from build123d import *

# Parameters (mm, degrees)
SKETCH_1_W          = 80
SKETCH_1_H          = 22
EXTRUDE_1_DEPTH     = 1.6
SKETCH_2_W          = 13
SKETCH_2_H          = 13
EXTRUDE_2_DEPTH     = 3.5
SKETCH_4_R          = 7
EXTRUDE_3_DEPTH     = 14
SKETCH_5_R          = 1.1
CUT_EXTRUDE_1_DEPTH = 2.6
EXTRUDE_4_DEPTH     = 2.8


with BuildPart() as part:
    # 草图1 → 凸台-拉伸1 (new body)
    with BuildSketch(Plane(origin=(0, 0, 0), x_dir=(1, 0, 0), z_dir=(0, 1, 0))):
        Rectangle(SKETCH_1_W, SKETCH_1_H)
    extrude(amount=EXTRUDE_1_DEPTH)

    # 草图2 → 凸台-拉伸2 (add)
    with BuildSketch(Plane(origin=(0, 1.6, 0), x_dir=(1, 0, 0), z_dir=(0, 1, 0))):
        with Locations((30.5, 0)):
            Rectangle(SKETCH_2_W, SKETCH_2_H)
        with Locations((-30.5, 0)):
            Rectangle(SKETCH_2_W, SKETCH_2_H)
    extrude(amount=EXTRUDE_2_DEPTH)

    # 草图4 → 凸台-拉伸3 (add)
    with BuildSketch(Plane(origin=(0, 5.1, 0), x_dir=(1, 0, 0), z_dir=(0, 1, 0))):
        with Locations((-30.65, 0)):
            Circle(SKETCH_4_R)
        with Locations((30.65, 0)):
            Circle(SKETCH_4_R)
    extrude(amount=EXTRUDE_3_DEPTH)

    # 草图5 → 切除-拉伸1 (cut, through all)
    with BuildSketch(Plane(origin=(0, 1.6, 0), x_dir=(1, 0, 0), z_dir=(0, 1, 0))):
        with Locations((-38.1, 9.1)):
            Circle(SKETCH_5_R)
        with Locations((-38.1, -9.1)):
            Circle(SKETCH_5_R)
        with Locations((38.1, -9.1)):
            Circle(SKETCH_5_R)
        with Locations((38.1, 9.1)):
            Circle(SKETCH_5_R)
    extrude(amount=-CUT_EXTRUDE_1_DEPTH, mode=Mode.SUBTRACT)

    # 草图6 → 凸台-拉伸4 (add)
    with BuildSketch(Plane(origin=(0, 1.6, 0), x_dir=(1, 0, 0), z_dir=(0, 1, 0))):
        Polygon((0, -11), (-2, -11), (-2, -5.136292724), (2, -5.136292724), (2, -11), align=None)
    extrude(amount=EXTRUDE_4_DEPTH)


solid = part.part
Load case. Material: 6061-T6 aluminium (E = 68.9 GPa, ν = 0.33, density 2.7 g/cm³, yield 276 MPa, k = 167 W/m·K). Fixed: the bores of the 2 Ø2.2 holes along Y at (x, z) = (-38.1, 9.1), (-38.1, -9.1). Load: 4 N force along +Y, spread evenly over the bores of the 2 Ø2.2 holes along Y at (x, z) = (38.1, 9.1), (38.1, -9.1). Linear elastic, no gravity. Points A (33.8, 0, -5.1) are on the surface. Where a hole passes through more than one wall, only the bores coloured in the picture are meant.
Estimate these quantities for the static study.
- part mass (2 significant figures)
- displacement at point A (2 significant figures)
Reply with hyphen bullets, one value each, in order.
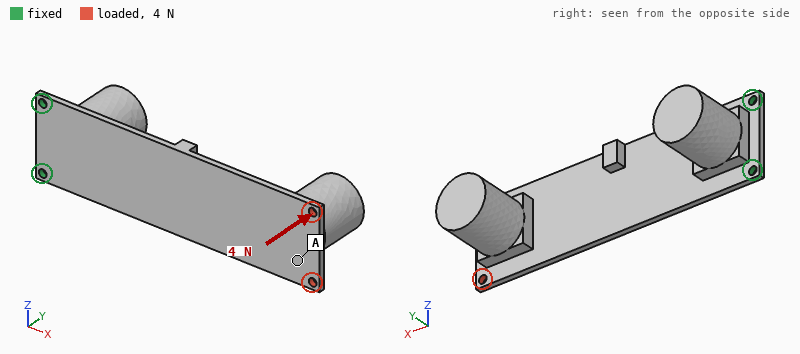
- 23 g
- 0.72 mm
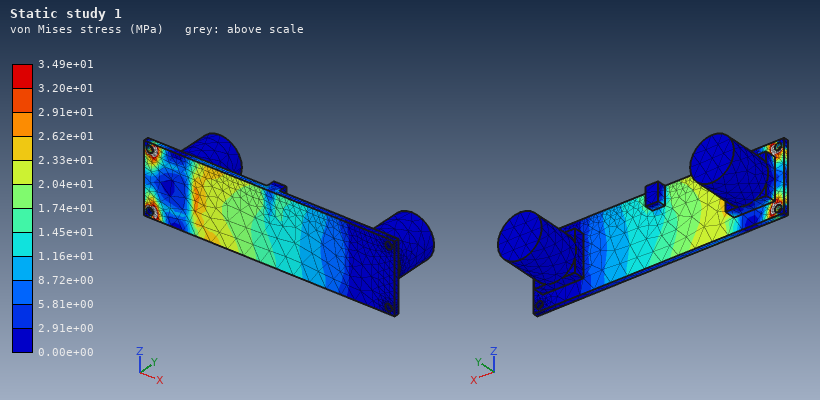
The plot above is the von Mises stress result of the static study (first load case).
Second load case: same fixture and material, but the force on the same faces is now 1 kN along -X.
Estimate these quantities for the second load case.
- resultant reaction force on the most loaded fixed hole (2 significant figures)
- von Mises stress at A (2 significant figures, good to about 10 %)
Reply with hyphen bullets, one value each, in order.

- 520 N
- 25 MPa
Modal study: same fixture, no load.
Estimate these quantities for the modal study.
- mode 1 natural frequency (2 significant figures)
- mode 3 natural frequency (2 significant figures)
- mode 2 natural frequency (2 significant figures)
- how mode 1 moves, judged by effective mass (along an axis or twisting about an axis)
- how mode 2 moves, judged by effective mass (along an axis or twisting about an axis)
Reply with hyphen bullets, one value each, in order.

- 130 Hz
- 870 Hz
- 630 Hz
- along Y
- along Z
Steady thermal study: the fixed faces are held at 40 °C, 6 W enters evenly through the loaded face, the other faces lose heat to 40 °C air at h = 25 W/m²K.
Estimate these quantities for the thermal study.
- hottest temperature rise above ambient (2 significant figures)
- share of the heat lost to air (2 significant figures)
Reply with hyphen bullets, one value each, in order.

- 51 K
- 48 %
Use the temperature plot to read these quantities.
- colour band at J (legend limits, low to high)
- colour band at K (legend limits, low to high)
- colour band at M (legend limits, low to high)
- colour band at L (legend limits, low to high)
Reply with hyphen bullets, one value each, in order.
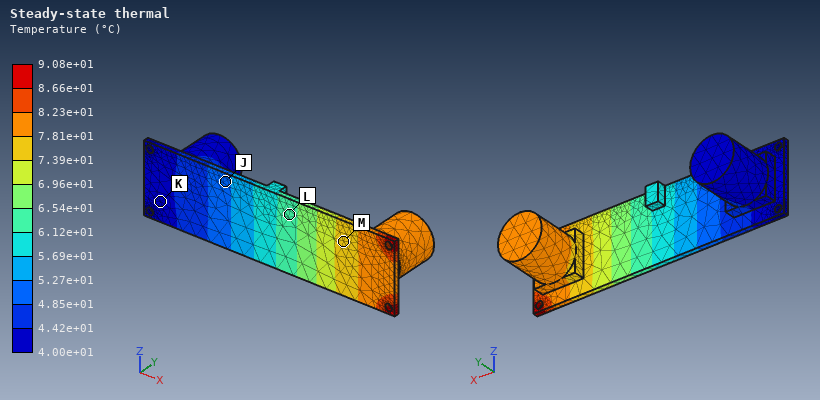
- 4.85e+01 to 5.27e+01 °C
- 4.00e+01 to 4.42e+01 °C
- 7.39e+01 to 7.81e+01 °C
- 6.12e+01 to 6.54e+01 °C
